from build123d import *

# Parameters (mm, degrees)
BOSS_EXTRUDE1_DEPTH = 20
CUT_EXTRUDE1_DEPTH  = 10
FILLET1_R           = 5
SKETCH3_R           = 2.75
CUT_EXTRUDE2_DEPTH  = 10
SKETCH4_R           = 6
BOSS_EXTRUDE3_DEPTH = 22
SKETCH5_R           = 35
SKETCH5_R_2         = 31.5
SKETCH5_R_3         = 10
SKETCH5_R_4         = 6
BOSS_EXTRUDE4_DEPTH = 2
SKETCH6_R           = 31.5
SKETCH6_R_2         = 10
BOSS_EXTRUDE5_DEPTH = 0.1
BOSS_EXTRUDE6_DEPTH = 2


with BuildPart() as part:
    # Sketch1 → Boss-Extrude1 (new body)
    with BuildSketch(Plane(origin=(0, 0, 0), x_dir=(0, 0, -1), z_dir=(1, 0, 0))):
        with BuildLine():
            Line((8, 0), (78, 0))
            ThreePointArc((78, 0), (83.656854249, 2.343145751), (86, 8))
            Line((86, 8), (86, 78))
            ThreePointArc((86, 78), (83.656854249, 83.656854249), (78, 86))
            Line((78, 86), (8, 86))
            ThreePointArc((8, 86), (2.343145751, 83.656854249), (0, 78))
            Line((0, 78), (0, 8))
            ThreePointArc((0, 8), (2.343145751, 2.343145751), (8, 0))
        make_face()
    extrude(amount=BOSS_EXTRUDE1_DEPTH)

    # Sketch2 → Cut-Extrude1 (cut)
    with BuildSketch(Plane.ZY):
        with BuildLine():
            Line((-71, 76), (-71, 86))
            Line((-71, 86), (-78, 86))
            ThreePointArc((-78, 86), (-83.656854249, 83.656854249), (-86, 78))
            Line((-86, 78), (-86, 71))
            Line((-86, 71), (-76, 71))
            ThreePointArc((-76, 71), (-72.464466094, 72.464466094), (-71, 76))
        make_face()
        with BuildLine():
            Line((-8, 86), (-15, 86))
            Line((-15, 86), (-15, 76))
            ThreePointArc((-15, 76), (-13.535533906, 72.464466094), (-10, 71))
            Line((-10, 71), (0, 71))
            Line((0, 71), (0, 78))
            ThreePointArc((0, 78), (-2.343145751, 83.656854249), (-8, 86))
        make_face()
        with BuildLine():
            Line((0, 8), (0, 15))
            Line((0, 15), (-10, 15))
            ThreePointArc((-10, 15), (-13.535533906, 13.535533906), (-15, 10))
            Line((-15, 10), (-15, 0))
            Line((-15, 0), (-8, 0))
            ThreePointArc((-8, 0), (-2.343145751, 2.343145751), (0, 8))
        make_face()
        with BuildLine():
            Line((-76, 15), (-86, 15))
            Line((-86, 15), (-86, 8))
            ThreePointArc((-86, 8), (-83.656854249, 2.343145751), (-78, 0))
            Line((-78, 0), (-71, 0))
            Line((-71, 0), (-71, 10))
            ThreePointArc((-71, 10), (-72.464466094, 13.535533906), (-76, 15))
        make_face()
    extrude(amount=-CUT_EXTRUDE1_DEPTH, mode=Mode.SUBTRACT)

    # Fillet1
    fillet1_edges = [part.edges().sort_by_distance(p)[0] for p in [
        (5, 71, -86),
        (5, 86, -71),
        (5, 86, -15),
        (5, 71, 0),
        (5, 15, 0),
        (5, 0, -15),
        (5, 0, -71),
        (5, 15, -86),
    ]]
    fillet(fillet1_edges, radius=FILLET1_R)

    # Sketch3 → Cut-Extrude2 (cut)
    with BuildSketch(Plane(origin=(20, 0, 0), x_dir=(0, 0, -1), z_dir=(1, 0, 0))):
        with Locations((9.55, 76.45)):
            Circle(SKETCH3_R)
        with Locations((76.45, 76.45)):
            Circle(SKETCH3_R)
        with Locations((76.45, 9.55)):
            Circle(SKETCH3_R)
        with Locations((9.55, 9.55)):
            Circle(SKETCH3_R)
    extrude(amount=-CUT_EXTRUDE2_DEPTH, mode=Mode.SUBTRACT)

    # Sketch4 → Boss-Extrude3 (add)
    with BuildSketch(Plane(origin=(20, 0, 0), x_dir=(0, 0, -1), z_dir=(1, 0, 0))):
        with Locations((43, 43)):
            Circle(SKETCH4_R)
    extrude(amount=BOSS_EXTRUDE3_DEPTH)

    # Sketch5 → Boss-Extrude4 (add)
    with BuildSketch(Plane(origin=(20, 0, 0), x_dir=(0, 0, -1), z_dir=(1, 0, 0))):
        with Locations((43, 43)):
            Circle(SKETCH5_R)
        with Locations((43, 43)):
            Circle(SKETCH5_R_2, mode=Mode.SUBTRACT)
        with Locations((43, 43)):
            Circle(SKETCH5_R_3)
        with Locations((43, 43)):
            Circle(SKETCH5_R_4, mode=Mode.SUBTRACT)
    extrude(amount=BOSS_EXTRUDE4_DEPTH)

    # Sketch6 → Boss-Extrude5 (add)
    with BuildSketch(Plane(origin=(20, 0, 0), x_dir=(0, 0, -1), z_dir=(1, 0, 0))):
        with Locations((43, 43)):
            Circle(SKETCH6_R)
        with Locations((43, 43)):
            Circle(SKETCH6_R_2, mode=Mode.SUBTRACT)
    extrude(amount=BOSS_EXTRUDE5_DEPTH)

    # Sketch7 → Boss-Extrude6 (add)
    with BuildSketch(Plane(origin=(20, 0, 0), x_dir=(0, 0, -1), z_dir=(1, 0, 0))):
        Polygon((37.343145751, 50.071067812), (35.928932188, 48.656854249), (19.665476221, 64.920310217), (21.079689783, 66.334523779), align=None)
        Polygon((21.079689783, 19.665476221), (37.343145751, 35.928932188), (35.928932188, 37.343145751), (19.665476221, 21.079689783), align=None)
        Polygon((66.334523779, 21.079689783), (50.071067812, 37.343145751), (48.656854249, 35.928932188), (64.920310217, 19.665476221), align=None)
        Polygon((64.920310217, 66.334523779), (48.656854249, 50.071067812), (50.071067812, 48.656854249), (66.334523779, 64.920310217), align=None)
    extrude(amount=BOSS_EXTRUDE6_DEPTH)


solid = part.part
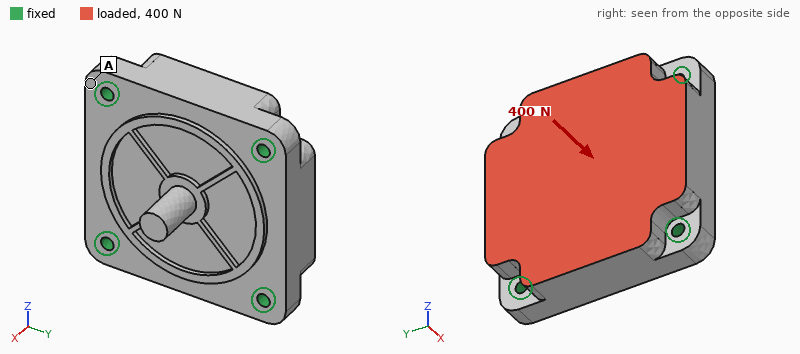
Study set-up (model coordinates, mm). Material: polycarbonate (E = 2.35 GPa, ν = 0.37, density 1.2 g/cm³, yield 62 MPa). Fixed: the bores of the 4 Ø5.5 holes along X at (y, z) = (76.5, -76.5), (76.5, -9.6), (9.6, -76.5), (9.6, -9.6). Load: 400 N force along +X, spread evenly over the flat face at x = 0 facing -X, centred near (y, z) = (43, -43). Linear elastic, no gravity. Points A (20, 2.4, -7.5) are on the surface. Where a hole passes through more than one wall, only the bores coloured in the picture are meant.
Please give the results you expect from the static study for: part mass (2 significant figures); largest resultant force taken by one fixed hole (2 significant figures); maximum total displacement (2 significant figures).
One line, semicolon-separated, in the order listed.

170 g; 110 N; 13 µm
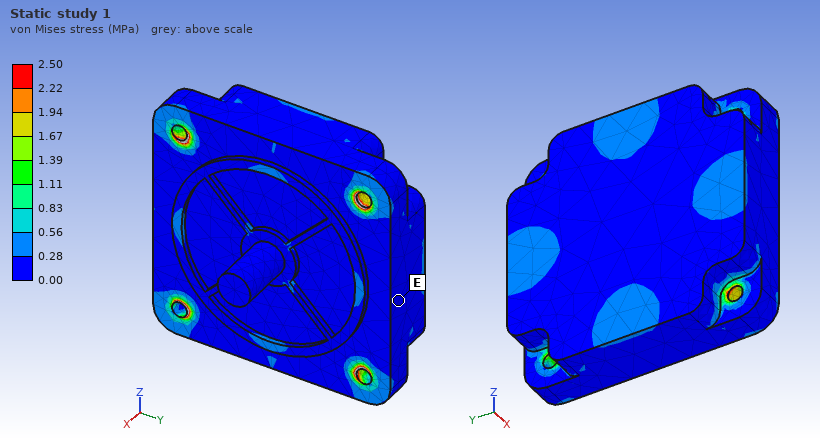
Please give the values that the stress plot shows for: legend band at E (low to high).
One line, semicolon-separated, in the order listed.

0.00 to 0.28 MPa
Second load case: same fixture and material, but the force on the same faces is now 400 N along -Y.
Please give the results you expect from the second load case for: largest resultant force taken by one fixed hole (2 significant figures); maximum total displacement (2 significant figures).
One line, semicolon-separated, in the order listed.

110 N; 9.6 µm
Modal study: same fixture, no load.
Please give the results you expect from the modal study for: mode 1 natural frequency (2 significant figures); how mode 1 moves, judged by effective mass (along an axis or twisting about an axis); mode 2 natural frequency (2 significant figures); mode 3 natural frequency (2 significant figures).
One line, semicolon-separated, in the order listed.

2400 Hz; along X; 3400 Hz; 3400 Hz
